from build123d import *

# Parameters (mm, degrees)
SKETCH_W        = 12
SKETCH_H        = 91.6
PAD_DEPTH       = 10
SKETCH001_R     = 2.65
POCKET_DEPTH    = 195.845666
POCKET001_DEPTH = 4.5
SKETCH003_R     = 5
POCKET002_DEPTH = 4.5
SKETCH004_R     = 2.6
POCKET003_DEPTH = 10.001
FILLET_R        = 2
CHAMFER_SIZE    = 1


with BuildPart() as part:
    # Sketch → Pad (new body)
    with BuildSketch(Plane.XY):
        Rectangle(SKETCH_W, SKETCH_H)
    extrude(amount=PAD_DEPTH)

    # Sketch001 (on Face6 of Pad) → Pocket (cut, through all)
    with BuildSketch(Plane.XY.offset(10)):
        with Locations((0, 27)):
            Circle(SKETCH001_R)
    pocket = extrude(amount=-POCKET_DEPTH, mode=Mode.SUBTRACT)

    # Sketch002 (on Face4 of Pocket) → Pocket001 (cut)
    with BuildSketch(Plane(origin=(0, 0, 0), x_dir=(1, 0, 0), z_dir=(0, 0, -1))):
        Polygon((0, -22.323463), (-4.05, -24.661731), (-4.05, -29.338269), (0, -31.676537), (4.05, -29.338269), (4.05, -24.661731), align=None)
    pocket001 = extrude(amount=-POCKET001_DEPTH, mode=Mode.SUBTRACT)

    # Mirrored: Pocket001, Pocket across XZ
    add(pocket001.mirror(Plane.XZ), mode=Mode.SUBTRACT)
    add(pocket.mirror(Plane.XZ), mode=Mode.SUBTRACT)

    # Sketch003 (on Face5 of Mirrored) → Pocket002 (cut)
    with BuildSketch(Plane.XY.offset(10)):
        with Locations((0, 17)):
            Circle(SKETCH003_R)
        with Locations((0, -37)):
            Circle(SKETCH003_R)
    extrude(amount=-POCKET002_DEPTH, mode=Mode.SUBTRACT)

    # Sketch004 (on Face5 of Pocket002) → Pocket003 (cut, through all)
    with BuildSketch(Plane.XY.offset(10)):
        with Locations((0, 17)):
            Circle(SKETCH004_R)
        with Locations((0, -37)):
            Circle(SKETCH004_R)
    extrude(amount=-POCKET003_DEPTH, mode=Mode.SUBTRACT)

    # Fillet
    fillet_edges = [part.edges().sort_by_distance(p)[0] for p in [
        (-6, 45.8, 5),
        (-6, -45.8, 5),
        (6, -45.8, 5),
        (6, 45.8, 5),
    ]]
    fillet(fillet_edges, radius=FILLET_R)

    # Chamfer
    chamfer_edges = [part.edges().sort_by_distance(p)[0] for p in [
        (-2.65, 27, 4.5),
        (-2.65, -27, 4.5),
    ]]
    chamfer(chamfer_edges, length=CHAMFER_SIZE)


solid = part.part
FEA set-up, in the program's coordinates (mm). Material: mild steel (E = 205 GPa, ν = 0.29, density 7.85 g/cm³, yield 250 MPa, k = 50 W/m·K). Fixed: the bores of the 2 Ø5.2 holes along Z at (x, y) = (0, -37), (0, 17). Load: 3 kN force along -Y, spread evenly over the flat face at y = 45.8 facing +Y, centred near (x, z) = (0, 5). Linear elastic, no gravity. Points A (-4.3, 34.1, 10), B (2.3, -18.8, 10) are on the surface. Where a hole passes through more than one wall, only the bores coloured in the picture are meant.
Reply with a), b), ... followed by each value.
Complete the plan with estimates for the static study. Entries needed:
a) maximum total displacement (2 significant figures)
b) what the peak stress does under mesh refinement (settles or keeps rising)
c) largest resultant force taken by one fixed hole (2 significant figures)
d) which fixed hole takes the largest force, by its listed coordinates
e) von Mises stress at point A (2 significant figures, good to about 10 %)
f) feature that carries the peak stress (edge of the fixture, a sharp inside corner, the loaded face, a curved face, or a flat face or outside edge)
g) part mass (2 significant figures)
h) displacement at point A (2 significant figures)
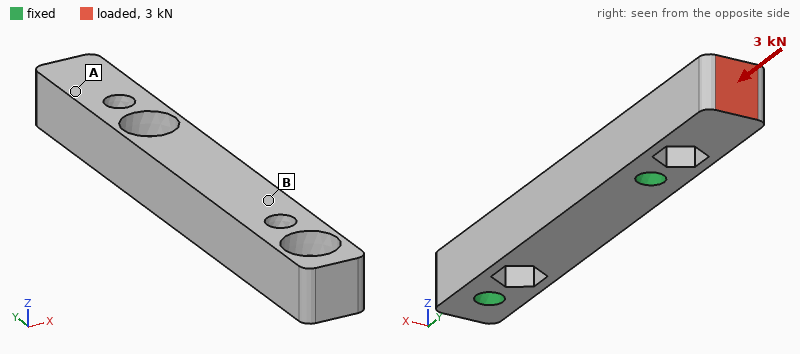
a) 10.0 µm
b) keeps rising
c) 2.8 kN
d) (0, 17)
e) 30 MPa
f) a sharp inside corner
g) 73 g
h) 7.5 µm
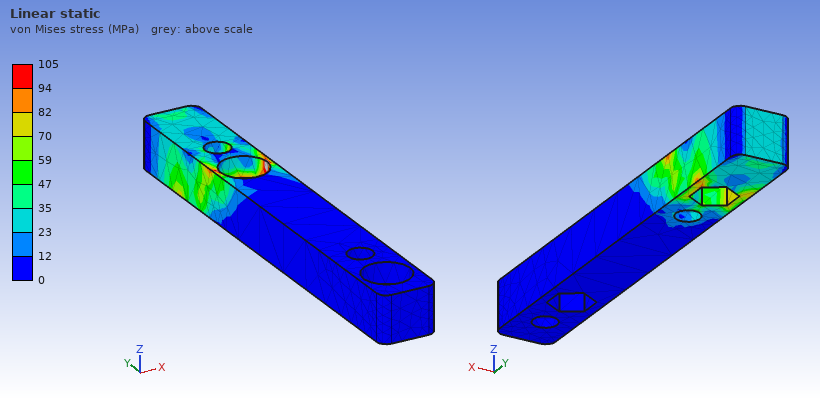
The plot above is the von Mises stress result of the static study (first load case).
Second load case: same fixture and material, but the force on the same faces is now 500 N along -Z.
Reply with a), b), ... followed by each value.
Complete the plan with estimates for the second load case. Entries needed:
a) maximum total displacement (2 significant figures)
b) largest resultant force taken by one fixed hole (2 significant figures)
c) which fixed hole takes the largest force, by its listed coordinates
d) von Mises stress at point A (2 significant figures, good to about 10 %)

a) 54 µm
b) 580 N
c) (0, 17)
d) 35 MPa
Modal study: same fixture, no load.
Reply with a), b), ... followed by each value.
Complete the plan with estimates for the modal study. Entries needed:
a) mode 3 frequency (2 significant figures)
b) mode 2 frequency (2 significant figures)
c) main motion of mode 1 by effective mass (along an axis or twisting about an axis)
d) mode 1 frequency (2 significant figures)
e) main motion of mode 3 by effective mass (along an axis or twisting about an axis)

a) 13 kHz
b) 7500 Hz
c) along Z
d) 5800 Hz
e) along Z
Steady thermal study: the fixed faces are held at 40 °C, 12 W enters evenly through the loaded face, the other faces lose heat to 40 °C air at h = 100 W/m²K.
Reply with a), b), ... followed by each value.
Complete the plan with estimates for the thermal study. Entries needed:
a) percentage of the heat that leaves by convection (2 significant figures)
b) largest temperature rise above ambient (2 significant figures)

a) 38 %
b) 62 K
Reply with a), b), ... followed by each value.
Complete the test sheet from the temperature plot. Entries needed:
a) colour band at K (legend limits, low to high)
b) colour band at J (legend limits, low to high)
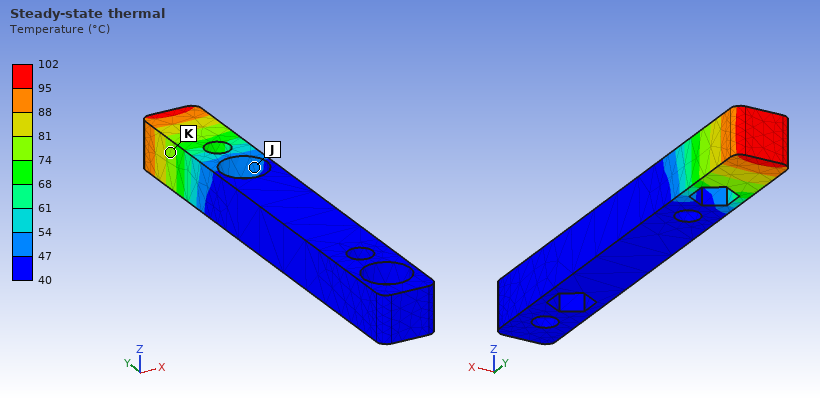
a) 74 to 81 °C
b) 47 to 54 °C
